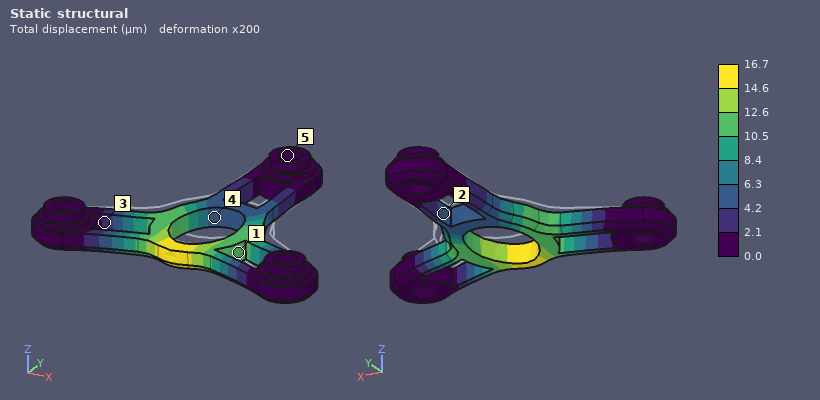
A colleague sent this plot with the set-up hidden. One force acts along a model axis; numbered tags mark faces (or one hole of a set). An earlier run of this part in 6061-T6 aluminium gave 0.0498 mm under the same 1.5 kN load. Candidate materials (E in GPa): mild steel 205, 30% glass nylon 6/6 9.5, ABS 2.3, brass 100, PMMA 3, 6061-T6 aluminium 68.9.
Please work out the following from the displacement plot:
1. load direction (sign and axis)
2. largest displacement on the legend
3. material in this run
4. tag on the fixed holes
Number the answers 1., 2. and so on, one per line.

1. -Y
2. 16.7 µm
3. mild steel
4. 5
